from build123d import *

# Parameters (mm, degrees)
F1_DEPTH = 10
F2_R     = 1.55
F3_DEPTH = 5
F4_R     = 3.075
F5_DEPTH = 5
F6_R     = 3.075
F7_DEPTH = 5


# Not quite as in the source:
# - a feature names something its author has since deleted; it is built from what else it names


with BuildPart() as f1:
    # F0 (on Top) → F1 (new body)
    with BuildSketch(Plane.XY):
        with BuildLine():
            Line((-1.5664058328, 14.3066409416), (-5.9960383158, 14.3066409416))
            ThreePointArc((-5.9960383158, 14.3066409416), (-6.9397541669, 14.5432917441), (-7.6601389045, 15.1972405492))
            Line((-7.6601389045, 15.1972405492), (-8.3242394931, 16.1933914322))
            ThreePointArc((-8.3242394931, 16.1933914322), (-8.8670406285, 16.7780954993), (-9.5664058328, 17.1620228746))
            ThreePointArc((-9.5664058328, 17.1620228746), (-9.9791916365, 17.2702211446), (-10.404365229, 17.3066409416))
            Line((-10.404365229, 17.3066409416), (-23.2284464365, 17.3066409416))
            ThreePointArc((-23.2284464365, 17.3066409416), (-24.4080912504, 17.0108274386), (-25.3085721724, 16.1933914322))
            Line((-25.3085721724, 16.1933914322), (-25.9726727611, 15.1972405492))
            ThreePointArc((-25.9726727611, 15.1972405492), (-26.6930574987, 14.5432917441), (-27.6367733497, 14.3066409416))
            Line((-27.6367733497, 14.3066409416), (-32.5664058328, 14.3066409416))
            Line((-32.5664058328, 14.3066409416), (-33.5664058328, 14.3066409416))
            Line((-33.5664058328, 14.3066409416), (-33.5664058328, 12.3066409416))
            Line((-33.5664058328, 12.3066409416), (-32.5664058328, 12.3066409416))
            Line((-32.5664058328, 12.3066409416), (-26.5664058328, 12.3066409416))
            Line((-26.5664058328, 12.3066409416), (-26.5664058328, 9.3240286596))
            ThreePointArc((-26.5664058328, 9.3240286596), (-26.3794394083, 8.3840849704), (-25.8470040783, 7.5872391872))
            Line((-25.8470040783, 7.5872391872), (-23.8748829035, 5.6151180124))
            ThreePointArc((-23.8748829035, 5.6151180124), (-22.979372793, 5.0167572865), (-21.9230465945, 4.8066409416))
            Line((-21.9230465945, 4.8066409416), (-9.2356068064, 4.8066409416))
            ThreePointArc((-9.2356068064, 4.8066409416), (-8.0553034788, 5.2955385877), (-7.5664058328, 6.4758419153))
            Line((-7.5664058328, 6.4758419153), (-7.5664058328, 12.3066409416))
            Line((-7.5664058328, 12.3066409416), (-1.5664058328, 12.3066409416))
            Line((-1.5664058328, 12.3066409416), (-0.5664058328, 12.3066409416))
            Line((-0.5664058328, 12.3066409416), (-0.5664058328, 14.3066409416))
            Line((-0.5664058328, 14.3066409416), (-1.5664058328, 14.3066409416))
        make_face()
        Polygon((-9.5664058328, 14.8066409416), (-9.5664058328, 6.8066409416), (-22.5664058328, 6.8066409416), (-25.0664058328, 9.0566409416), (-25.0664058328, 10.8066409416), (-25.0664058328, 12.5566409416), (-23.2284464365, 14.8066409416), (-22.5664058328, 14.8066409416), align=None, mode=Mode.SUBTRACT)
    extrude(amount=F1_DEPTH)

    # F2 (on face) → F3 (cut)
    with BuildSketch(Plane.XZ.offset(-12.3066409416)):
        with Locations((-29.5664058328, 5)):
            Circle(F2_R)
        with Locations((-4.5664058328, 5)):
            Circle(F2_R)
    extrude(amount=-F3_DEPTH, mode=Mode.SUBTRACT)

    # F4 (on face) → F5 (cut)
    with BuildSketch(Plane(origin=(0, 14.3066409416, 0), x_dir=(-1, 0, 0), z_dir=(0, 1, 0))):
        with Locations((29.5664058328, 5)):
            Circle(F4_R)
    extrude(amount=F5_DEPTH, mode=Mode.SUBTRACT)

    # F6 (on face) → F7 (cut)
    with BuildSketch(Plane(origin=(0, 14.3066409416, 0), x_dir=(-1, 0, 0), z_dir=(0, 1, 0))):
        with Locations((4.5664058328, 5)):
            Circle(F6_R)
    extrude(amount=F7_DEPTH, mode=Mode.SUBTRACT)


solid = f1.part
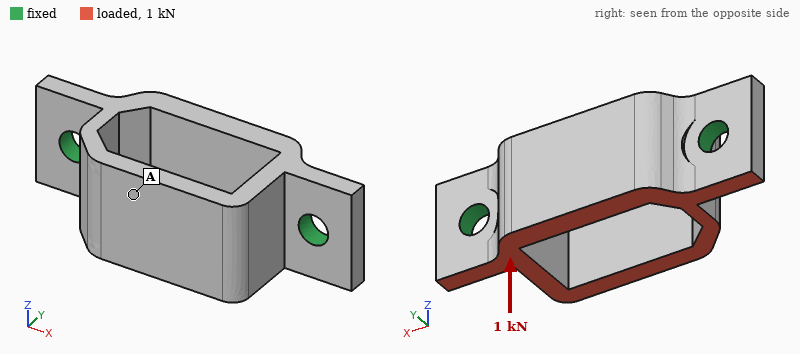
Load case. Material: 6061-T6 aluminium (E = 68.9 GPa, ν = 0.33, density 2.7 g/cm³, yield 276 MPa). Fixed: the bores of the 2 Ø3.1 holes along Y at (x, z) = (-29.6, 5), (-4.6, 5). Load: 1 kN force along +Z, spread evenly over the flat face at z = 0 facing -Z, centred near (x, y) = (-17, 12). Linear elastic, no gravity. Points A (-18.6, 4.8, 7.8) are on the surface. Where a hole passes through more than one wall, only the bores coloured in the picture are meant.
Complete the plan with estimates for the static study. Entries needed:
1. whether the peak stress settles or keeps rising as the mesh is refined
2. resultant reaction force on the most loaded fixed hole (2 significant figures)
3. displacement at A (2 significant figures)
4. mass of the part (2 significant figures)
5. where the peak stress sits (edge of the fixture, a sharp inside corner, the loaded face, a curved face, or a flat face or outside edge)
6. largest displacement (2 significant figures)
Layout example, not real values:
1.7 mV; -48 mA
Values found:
keeps rising; 520 N; 28 µm; 3.6 g; edge of the fixture; 30 µm
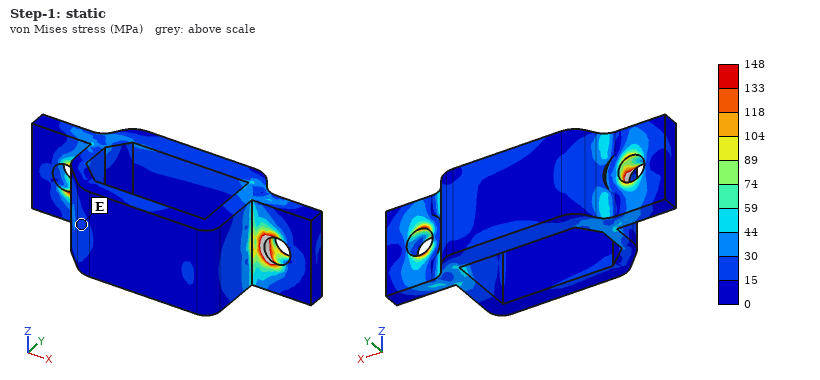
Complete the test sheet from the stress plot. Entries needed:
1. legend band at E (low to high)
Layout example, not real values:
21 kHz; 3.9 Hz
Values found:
15 to 30 MPa
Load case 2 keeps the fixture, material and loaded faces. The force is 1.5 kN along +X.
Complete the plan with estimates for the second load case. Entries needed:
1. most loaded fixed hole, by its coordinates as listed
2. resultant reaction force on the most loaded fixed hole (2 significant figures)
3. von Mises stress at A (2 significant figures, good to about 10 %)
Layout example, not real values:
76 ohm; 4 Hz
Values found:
(-4.6, 5); 860 N; 18 MPa
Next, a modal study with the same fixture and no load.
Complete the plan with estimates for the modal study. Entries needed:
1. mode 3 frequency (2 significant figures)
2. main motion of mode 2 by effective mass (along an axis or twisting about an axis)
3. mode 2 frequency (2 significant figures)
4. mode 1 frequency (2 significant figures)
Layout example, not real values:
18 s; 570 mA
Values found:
26 kHz; along X; 17 kHz; 14 kHz
